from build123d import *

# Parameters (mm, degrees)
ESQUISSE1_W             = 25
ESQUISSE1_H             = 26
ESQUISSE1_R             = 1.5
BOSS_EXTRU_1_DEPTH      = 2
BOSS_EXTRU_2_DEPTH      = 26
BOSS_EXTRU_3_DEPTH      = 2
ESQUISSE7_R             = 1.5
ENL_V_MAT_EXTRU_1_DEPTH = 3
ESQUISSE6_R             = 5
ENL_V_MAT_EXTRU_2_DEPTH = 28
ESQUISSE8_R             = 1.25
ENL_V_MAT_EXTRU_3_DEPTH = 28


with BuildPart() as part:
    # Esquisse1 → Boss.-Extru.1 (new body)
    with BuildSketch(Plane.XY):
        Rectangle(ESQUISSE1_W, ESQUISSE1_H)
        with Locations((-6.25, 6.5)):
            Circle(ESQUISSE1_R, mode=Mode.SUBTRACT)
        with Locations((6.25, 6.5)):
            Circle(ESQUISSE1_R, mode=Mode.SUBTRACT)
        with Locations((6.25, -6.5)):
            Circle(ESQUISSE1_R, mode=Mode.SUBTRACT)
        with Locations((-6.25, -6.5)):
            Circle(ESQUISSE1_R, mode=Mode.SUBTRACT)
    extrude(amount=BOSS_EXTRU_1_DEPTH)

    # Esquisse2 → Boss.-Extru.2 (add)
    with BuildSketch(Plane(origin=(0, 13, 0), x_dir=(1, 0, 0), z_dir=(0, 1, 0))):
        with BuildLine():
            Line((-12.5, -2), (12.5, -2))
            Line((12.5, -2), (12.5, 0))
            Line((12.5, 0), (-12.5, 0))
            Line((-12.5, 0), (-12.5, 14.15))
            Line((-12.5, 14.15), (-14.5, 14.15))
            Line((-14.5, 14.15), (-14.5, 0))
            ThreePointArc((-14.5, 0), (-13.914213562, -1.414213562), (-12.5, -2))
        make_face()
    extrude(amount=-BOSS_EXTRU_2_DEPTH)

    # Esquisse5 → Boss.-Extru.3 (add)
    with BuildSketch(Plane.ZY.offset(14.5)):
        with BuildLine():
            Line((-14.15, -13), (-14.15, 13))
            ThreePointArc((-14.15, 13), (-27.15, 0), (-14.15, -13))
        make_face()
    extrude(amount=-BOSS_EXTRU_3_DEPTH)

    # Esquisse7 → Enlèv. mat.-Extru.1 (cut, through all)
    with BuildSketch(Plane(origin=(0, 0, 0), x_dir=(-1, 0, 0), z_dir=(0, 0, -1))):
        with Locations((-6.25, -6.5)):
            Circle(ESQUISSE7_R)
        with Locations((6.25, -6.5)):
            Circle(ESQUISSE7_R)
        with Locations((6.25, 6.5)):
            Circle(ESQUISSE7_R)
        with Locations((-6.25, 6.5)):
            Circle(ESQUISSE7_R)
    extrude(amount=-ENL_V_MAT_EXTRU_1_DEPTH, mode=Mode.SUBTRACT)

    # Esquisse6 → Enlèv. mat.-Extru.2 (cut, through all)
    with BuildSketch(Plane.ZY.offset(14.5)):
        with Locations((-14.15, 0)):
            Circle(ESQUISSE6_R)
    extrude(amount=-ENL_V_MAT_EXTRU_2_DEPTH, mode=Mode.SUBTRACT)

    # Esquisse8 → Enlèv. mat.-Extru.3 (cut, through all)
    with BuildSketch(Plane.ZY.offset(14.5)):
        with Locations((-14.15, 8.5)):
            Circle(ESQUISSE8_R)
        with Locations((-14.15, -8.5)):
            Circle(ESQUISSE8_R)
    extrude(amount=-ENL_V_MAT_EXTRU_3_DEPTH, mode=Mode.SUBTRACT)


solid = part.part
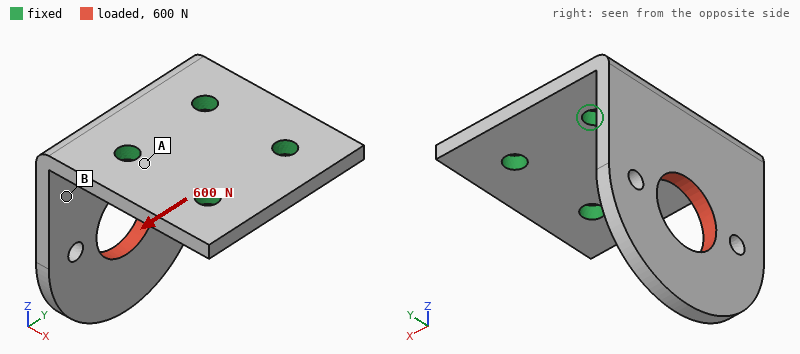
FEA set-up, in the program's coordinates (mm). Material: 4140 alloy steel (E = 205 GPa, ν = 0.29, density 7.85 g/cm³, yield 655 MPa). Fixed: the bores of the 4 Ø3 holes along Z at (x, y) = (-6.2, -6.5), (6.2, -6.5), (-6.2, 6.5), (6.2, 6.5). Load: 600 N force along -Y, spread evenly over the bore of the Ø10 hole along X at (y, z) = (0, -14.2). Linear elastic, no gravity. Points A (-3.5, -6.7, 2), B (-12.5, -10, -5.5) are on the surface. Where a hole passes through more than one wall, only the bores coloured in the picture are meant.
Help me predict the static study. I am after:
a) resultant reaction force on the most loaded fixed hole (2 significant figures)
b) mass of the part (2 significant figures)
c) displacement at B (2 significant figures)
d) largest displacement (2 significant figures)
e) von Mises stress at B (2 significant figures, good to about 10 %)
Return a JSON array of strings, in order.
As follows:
["710 N", "19 g", "39 µm", "92 µm", "82 MPa"]
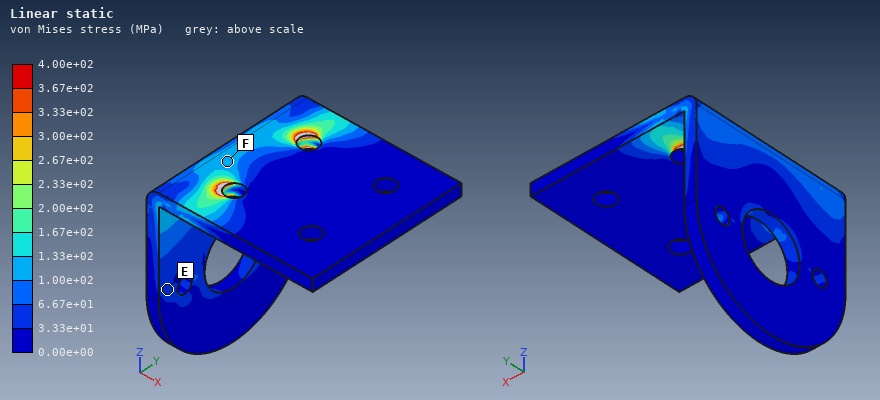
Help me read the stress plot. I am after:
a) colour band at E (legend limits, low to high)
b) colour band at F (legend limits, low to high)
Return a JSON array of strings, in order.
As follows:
["3.33e+01 to 6.67e+01 MPa", "1.00e+02 to 1.33e+02 MPa"]
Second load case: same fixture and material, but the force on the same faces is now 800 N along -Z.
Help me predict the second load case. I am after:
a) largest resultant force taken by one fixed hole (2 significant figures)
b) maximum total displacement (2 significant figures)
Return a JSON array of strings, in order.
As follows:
["440 N", "0.15 mm"]
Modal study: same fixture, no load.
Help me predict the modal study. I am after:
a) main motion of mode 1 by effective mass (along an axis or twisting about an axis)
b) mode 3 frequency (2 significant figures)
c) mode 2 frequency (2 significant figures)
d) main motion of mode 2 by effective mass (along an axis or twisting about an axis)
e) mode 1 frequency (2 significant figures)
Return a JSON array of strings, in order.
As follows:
["along X", "6800 Hz", "4800 Hz", "along Y", "1900 Hz"]
